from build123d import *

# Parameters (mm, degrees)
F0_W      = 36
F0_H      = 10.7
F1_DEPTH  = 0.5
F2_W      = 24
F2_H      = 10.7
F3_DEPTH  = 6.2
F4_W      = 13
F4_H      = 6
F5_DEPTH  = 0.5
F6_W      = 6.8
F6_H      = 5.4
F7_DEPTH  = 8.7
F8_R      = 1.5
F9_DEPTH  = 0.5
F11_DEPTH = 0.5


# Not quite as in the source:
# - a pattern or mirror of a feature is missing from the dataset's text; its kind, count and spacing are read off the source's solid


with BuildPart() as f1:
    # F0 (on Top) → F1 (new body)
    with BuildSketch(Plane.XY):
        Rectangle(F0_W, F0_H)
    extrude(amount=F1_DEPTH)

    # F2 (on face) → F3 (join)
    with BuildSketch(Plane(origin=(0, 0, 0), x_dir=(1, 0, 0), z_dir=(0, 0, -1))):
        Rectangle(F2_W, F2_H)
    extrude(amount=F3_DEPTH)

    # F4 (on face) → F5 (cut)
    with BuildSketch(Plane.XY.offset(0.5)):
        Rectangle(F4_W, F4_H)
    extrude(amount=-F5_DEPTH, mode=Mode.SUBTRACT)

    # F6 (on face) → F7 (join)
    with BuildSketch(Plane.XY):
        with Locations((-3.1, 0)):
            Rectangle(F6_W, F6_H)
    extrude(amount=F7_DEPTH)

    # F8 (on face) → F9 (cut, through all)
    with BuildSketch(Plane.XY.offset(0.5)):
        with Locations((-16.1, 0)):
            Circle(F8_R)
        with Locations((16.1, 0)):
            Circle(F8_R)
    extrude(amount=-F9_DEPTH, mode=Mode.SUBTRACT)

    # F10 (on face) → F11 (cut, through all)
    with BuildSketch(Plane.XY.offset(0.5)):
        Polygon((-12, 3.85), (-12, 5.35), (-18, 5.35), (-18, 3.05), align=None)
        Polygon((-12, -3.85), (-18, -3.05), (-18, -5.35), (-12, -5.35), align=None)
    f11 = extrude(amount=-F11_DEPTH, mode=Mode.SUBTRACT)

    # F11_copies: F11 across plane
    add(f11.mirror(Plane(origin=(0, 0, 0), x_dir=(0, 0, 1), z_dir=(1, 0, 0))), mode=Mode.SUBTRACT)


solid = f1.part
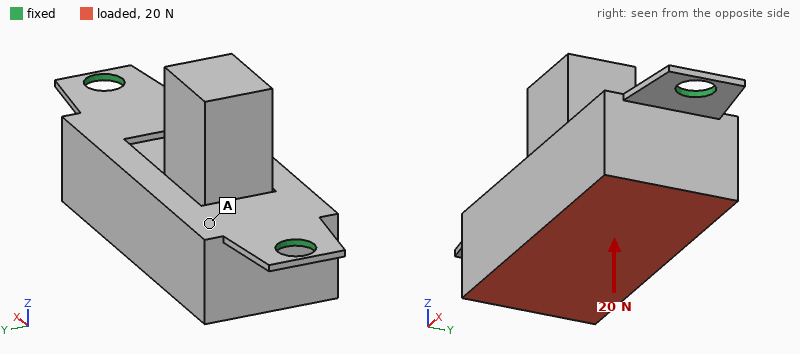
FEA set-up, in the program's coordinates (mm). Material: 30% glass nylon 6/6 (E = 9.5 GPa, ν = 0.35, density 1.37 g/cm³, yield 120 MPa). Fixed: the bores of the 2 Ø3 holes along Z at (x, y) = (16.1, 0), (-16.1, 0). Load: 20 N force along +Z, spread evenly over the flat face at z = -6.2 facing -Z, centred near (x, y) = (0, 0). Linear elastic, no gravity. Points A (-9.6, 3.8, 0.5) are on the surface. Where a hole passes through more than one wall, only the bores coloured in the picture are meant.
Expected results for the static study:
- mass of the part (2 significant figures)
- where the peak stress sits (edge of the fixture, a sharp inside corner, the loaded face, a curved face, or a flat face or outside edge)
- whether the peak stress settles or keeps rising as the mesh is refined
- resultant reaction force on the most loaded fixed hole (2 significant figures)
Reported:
2.8 g
edge of the fixture
keeps rising
13 N
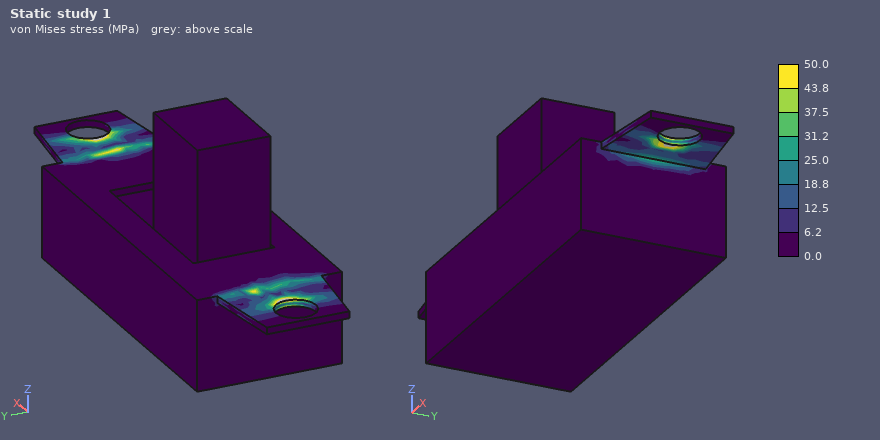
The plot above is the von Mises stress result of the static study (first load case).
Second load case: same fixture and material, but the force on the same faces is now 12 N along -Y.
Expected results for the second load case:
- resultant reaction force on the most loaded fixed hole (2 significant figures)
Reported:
6.0 N
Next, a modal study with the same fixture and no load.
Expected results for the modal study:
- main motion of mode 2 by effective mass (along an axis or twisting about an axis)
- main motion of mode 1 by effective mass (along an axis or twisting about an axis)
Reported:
along Z
along Y
